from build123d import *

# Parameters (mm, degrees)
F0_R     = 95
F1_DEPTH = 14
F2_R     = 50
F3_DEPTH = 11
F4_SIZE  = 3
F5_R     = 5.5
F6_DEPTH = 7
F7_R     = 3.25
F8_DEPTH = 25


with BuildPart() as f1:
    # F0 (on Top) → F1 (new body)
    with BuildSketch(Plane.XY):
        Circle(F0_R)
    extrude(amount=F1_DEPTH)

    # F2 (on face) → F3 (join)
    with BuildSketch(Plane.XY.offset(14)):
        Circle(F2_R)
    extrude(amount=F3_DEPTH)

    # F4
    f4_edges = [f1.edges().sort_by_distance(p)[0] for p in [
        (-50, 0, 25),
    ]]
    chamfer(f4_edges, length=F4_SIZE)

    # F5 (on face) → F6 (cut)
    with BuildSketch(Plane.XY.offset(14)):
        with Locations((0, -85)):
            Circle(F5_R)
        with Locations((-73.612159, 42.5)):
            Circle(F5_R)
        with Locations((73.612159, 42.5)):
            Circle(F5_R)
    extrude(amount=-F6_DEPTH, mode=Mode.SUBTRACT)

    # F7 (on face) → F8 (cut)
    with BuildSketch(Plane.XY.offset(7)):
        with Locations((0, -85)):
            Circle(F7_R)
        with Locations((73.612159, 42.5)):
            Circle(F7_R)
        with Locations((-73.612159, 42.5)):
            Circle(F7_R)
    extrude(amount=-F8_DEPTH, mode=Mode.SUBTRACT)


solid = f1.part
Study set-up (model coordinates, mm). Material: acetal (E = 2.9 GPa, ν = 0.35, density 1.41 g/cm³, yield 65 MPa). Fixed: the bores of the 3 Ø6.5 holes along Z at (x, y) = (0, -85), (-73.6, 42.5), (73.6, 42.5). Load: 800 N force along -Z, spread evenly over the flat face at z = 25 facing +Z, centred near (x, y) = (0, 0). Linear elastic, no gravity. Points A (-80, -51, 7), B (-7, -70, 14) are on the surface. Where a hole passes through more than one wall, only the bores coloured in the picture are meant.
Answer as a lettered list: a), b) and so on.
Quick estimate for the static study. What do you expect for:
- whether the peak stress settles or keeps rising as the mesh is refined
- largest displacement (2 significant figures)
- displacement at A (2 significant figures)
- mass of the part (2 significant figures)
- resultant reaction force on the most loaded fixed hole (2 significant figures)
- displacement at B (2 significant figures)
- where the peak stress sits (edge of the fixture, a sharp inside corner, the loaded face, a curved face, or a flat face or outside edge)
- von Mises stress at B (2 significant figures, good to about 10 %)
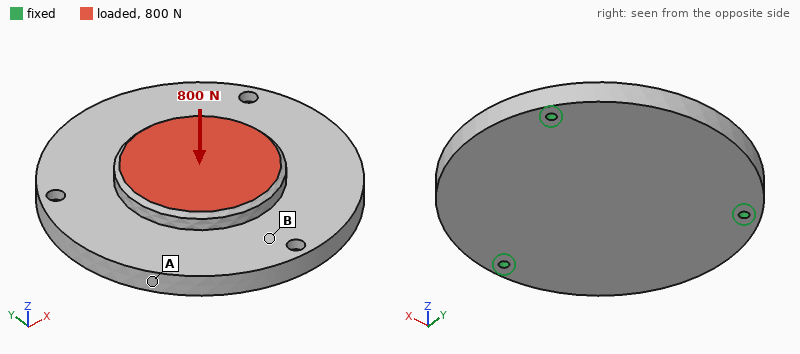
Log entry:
a) keeps rising
b) 0.12 mm
c) 0.097 mm
d) 680 g
e) 400 N
f) 0.049 mm
g) edge of the fixture
h) 1.4 MPa
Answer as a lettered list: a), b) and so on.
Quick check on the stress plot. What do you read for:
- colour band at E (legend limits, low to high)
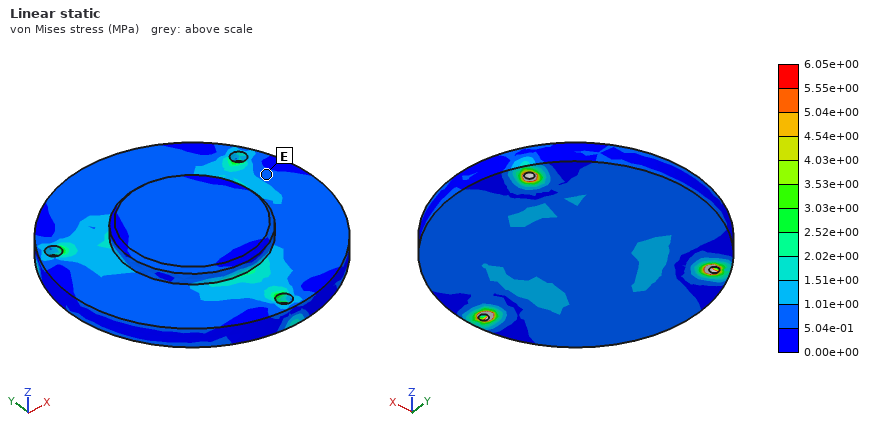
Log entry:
a) 5.04e-01 to 1.01e+00 MPa
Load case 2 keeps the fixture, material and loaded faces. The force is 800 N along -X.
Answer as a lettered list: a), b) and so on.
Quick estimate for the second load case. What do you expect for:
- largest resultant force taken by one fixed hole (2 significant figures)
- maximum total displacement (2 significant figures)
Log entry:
a) 350 N
b) 70 µm
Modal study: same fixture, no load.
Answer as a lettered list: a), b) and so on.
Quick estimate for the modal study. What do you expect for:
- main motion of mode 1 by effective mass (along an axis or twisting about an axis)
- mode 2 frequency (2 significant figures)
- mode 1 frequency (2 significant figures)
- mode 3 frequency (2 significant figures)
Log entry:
a) along Z
b) 620 Hz
c) 590 Hz
d) 620 Hz
